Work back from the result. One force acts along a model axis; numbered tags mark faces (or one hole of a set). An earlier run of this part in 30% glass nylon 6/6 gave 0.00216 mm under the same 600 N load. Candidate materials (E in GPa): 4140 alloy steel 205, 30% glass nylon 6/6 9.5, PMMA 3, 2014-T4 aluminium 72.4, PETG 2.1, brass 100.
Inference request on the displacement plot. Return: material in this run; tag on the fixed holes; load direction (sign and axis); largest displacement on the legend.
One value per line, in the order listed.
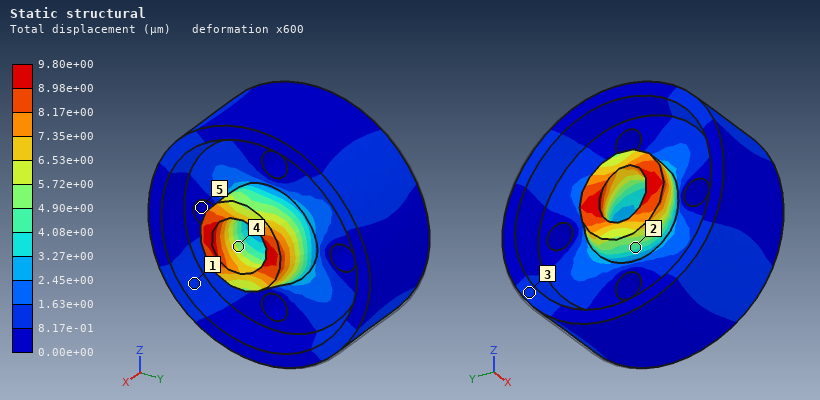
PETG
5
-Y
9.80e+00 µm
